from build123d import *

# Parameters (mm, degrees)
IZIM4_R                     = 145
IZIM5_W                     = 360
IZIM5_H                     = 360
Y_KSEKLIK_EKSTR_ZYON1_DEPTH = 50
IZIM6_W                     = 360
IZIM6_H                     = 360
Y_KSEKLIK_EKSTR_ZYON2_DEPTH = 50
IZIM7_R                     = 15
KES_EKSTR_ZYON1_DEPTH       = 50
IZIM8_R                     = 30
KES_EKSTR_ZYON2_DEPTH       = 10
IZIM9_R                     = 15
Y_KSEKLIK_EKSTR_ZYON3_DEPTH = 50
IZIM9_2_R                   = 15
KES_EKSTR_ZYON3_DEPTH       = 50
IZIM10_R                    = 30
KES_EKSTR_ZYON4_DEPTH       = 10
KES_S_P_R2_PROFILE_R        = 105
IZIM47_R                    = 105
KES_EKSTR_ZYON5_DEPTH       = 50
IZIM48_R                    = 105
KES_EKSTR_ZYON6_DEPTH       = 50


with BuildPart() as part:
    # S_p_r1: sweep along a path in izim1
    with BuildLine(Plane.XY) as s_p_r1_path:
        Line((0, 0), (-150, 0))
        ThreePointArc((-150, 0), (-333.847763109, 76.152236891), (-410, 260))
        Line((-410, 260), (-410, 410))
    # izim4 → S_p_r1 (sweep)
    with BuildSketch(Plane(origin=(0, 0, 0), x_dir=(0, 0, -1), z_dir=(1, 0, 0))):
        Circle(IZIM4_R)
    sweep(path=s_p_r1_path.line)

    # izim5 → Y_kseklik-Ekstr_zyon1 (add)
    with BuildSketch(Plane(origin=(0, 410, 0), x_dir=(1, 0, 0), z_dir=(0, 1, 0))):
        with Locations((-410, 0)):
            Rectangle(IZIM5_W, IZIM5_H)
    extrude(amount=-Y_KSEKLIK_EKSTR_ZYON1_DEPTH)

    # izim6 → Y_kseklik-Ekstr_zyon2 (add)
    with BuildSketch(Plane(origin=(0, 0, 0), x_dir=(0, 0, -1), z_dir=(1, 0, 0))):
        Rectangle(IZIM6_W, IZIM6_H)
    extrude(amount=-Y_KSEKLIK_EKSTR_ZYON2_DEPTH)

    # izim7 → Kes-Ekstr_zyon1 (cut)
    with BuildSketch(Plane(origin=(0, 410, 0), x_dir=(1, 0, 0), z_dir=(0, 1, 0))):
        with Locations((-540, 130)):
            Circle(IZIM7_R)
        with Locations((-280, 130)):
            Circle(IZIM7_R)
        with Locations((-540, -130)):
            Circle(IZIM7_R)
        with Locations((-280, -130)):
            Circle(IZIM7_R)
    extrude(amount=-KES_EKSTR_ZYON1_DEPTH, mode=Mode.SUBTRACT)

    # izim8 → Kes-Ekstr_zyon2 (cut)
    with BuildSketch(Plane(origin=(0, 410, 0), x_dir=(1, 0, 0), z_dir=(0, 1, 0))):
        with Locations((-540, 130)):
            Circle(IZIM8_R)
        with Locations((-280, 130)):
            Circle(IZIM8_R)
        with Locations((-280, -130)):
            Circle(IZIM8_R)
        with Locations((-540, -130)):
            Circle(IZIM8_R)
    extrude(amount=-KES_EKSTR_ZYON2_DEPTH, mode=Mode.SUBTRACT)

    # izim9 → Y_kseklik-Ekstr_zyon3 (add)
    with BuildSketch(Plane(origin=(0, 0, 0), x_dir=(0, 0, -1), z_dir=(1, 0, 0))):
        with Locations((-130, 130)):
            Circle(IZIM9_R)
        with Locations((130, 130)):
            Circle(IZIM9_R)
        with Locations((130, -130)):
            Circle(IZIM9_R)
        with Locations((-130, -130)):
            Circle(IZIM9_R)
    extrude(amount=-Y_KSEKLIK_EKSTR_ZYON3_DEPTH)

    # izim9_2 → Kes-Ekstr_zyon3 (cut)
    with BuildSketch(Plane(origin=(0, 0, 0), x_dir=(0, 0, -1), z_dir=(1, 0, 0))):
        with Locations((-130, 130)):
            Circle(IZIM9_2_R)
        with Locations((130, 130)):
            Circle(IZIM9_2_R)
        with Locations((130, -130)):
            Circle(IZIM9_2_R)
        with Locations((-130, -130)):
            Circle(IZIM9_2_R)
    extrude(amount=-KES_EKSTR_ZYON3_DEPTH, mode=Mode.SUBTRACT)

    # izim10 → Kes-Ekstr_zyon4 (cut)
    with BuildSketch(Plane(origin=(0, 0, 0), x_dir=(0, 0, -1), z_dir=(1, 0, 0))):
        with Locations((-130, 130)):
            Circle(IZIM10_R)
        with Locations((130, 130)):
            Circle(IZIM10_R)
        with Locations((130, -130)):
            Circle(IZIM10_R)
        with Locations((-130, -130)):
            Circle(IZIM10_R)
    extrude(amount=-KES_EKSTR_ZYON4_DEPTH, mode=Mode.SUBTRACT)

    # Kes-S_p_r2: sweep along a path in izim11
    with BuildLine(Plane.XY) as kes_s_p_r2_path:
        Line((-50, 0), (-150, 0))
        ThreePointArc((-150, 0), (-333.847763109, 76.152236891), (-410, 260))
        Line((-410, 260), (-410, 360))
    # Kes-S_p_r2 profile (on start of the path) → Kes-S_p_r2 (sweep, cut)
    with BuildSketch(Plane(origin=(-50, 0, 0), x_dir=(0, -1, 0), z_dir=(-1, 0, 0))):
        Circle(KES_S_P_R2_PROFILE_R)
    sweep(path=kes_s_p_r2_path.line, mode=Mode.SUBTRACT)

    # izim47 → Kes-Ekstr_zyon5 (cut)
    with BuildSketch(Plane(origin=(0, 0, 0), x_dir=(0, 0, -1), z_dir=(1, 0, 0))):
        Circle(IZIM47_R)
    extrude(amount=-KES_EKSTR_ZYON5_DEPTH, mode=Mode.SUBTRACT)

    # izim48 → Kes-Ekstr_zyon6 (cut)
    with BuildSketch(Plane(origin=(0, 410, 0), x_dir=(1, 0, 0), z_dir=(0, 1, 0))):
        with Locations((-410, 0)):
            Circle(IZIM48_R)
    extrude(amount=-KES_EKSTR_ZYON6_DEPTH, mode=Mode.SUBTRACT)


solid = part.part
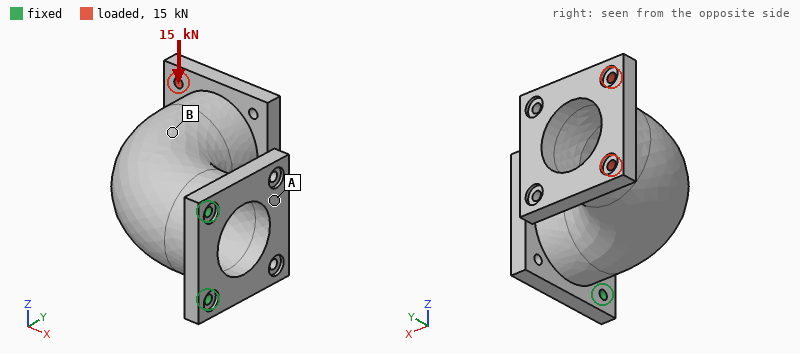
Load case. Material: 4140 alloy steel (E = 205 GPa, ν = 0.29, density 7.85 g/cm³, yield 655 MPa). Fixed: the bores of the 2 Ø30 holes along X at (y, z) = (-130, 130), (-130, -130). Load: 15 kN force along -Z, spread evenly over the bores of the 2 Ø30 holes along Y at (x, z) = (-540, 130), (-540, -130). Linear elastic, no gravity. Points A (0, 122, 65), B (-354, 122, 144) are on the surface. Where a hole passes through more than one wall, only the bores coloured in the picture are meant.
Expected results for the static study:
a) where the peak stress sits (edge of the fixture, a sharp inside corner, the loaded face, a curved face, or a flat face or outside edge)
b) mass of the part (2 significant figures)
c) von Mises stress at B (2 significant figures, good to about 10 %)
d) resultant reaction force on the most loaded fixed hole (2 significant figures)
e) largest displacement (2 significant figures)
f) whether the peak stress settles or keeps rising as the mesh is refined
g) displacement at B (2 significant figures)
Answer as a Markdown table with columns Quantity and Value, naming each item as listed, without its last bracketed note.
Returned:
| Quantity | Value |
|---|---|
| where the peak stress sits | edge of the fixture |
| mass of the part | 220 kg |
| von Mises stress at B | 4.2 MPa |
| resultant reaction force on the most loaded fixed hole | 42 kN |
| largest displacement | 0.13 mm |
| whether the peak stress settles or keeps rising as the mesh is refined | keeps rising |
| displacement at B | 0.059 mm |
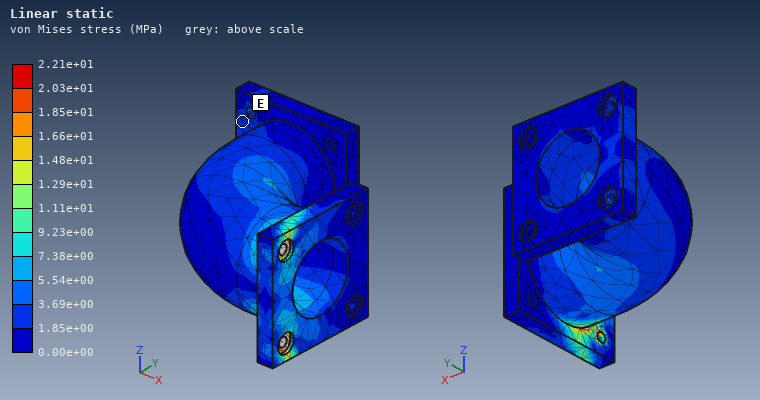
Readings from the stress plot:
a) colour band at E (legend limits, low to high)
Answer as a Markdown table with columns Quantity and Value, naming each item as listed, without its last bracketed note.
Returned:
| Quantity | Value |
|---|---|
| colour band at E | 1.85e+00 to 3.69e+00 MPa |
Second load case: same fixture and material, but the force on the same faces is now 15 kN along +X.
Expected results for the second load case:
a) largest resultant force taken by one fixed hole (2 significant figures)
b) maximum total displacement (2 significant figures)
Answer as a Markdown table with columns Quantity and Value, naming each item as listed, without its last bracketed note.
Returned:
| Quantity | Value |
|---|---|
| largest resultant force taken by one fixed hole | 7.5 kN |
| maximum total displacement | 0.78 mm |
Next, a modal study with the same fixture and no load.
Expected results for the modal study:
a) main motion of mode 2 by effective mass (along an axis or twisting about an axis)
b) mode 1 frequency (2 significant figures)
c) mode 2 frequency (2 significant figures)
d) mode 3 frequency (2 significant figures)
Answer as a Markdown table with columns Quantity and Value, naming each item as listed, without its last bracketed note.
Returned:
| Quantity | Value |
|---|---|
| main motion of mode 2 by effective mass | along Z |
| mode 1 frequency | 69 Hz |
| mode 2 frequency | 220 Hz |
| mode 3 frequency | 550 Hz |
